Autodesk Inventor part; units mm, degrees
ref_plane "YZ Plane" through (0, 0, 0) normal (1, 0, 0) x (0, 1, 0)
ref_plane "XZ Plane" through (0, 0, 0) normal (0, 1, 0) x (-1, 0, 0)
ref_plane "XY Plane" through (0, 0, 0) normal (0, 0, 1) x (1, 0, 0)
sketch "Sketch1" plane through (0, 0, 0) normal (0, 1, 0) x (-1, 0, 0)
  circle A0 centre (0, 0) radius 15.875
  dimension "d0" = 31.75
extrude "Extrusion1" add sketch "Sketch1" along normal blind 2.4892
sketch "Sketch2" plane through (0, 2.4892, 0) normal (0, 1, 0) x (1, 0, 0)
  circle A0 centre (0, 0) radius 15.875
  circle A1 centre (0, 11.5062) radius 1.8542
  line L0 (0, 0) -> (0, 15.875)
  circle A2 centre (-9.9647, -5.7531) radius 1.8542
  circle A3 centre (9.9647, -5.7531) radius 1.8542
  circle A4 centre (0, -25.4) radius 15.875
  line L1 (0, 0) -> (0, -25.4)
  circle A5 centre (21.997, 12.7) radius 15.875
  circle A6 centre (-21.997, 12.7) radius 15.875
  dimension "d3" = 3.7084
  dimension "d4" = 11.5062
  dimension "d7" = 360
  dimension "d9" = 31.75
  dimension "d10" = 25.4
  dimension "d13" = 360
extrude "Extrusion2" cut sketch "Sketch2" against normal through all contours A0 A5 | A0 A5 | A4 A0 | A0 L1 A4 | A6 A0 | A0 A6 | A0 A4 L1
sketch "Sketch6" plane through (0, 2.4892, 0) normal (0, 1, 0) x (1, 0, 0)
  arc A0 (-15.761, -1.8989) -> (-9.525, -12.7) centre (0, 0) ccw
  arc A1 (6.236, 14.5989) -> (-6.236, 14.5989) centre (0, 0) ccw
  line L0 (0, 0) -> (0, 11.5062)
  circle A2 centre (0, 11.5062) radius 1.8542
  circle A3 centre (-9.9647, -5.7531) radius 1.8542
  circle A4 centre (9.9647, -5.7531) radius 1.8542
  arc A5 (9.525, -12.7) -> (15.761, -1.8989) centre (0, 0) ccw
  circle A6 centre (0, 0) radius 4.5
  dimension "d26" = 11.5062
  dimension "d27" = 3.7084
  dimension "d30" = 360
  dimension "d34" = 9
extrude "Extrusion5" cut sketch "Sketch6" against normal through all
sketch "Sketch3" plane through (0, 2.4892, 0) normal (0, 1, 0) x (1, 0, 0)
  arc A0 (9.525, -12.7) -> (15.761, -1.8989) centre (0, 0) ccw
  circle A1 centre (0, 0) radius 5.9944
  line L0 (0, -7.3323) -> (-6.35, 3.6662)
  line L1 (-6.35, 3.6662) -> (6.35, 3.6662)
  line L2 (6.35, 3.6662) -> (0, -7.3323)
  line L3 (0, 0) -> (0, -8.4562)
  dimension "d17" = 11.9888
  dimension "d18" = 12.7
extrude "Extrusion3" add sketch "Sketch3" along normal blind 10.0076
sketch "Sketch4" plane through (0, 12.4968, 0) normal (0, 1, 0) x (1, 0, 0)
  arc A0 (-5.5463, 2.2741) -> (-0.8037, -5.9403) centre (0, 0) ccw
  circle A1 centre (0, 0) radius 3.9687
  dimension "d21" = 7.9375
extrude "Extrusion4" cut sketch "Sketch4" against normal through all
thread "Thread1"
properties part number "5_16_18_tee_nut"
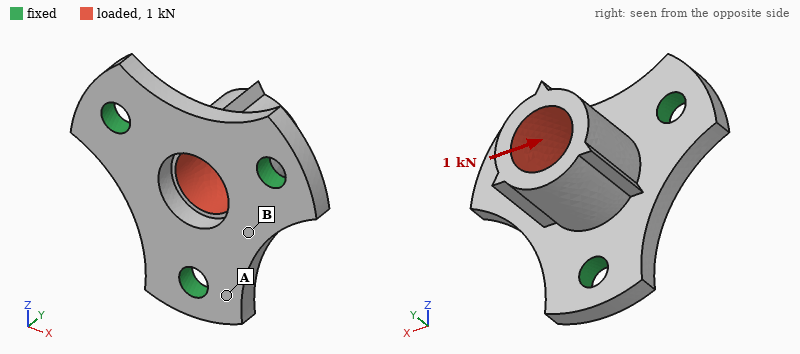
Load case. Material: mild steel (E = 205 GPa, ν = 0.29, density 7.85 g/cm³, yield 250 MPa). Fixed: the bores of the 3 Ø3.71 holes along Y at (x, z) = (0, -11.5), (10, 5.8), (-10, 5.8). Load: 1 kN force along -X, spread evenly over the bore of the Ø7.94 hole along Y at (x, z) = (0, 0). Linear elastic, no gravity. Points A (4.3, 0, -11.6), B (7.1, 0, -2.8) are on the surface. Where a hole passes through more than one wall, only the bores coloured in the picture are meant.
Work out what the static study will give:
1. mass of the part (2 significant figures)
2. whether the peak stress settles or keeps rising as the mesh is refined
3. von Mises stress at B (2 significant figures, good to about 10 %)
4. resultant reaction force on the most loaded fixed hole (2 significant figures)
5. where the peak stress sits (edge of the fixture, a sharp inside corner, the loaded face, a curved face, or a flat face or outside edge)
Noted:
14 g
keeps rising
52 MPa
540 N
edge of the fixture
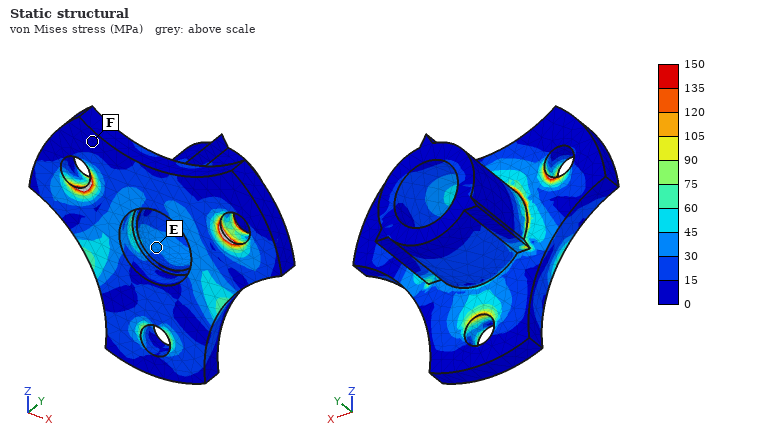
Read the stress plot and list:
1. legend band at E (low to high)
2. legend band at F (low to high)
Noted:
30 to 45 MPa
0 to 15 MPa
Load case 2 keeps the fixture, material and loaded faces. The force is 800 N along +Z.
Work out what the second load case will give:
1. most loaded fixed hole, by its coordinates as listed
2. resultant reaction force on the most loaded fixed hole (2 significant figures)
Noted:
(0, -11.5)
480 N
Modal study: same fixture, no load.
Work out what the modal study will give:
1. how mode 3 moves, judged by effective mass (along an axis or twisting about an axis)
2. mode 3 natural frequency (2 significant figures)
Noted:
along Y
28 kHz
